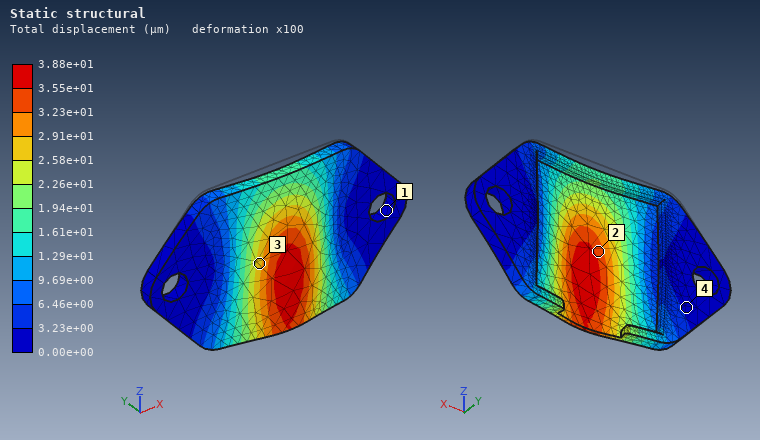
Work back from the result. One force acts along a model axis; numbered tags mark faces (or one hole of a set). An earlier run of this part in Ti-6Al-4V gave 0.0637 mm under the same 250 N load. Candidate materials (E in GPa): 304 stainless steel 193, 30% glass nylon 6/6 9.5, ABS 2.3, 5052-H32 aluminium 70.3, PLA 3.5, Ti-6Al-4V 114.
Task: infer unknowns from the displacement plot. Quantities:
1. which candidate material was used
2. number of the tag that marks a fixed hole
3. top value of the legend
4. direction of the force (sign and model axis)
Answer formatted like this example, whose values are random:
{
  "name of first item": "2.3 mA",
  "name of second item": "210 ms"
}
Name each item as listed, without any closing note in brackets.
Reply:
{
  "which candidate material was used": "304 stainless steel",
  "number of the tag that marks a fixed hole": "1",
  "top value of the legend": "3.88e+01 µm",
  "direction of the force": "-Y"
}
